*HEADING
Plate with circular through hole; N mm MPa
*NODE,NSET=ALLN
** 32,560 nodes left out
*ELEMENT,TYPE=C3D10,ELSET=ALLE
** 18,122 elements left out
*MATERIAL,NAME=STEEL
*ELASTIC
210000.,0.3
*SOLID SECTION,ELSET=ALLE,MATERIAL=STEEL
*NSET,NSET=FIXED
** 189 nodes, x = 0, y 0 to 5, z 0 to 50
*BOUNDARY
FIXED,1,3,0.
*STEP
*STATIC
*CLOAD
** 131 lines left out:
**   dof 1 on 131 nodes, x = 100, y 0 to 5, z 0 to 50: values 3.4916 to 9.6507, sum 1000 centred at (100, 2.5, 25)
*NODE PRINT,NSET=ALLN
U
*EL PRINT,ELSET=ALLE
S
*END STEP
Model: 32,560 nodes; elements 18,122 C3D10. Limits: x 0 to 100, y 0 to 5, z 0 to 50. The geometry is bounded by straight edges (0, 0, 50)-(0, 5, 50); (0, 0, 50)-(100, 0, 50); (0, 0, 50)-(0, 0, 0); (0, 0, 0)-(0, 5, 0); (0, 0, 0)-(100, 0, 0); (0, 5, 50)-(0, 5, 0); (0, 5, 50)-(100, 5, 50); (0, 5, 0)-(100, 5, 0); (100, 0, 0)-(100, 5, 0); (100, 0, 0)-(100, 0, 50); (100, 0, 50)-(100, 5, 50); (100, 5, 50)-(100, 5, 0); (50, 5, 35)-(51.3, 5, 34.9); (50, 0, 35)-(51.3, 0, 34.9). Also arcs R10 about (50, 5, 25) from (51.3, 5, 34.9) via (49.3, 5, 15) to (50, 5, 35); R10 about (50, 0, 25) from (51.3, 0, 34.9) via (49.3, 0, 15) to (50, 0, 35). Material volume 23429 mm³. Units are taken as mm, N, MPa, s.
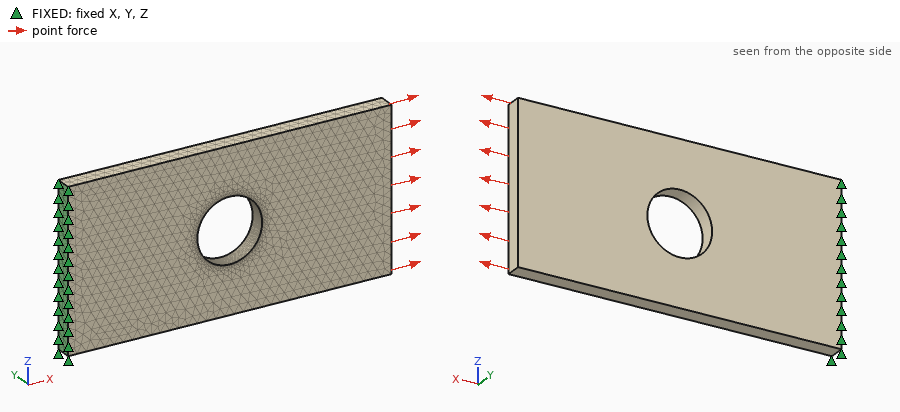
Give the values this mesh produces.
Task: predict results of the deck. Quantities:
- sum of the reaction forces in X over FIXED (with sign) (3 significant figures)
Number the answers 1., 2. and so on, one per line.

1. -1000 N
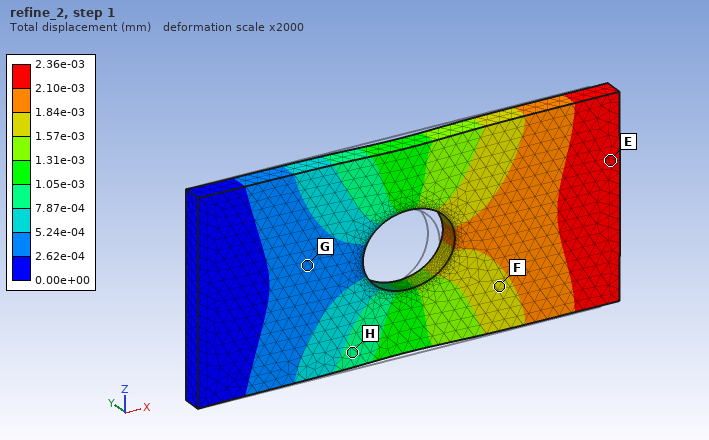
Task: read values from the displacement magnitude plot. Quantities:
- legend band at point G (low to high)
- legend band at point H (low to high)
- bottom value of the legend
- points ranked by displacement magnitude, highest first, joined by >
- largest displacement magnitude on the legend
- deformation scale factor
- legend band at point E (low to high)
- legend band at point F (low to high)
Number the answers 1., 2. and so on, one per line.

1. 2.62e-04 to 5.24e-04 mm
2. 7.87e-04 to 1.05e-03 mm
3. 0.00e+00 mm
4. E > F > H > G
5. 2.36e-03 mm
6. 2000
7. 2.10e-03 to 2.36e-03 mm
8. 1.57e-03 to 1.84e-03 mm
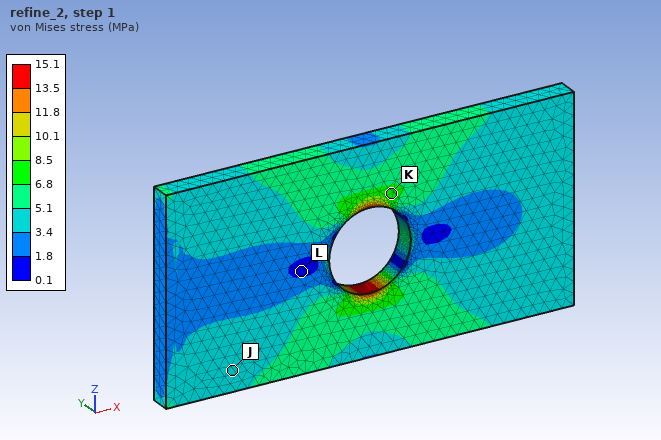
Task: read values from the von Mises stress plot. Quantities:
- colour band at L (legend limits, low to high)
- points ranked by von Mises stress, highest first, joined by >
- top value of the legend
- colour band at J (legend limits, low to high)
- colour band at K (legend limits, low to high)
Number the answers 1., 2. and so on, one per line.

1. 0.1 to 1.8 MPa
2. K > J > L
3. 15.1 MPa
4. 3.4 to 5.1 MPa
5. 6.8 to 8.5 MPa
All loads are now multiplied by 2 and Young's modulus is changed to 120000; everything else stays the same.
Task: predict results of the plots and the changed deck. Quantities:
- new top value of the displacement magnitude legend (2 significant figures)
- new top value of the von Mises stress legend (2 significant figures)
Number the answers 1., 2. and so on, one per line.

1. 0.0083 mm
2. 30 MPa
